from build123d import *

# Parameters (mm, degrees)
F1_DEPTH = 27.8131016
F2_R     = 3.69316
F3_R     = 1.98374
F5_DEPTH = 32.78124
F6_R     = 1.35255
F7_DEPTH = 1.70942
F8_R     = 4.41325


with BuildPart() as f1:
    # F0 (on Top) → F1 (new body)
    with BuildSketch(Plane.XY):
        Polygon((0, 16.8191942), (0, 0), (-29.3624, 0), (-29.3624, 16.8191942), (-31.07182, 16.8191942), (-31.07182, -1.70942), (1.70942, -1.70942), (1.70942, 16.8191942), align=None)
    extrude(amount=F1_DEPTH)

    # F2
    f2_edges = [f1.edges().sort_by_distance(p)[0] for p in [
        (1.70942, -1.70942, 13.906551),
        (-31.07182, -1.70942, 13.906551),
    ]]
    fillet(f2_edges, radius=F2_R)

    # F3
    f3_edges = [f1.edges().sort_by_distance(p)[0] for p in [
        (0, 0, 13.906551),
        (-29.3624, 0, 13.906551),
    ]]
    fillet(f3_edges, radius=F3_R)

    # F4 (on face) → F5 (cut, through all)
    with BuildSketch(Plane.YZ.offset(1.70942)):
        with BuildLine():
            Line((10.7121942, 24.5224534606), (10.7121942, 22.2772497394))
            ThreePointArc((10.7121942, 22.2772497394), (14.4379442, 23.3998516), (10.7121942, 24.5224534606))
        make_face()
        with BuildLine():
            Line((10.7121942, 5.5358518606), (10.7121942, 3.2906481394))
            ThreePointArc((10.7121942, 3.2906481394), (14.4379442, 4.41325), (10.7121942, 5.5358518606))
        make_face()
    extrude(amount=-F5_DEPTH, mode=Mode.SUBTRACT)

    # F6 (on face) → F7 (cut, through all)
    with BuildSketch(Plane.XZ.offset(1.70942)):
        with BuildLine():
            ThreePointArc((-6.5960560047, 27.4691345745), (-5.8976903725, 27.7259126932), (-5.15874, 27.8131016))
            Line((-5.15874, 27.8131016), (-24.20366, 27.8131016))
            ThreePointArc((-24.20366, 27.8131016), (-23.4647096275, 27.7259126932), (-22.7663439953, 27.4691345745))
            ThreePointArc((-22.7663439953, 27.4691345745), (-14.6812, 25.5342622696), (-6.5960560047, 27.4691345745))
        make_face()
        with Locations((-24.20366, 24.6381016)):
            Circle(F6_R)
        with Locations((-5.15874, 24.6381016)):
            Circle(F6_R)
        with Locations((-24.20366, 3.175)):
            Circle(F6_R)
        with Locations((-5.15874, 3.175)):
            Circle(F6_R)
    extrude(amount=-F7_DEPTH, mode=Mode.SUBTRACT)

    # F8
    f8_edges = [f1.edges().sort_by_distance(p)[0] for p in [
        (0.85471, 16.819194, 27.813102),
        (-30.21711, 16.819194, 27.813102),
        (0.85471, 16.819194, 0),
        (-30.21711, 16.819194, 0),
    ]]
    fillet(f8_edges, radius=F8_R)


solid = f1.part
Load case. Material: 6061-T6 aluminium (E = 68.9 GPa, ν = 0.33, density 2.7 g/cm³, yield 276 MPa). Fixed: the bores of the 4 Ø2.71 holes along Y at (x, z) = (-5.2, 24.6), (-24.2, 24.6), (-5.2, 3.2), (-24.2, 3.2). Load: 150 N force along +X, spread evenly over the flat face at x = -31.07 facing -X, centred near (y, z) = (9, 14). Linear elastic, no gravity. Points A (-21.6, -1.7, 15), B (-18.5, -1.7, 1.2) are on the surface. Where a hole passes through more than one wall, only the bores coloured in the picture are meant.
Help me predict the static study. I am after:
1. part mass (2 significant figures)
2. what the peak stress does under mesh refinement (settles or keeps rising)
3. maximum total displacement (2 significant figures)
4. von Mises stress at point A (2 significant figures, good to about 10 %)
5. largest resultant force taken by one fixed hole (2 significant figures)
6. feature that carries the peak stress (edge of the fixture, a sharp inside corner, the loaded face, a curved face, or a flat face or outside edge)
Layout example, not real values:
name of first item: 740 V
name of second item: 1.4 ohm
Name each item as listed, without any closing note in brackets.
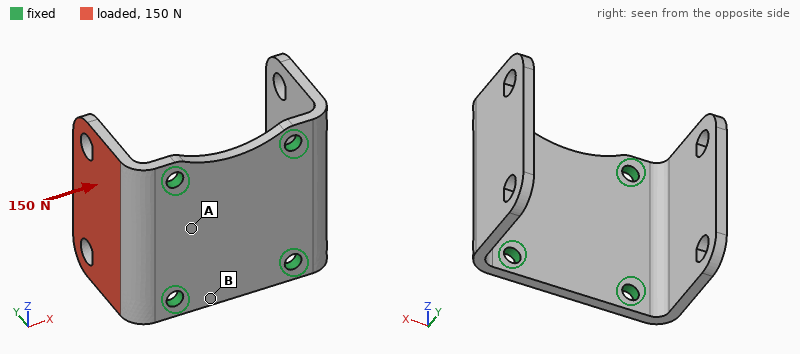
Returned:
part mass: 7.7 g
what the peak stress does under mesh refinement: keeps rising
maximum total displacement: 0.29 mm
von Mises stress at point A: 28 MPa
largest resultant force taken by one fixed hole: 56 N
feature that carries the peak stress: edge of the fixture
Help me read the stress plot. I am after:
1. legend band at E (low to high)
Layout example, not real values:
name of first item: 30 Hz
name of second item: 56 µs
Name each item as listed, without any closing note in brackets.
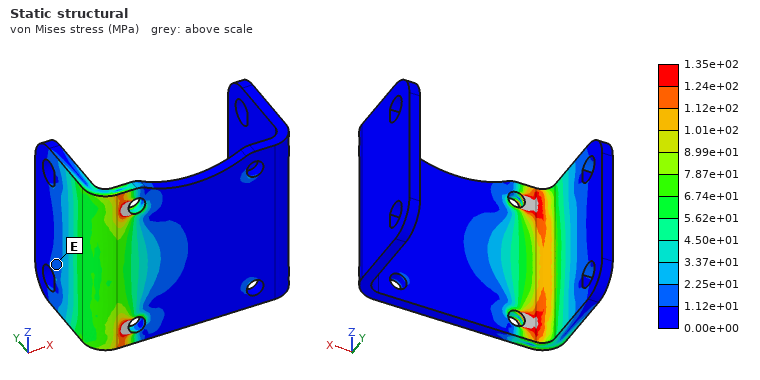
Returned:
legend band at E: 1.12e+01 to 2.25e+01 MPa
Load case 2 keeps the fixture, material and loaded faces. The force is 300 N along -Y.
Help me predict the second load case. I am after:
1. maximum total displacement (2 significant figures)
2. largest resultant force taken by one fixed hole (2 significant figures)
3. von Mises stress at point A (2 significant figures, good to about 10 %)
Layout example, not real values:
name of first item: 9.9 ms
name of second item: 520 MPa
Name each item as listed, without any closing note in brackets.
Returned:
maximum total displacement: 0.18 mm
largest resultant force taken by one fixed hole: 160 N
von Mises stress at point A: 25 MPa
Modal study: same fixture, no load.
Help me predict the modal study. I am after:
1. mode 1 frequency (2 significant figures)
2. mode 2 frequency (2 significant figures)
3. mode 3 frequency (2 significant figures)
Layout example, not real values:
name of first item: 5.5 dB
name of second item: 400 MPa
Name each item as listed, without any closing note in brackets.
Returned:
mode 1 frequency: 3300 Hz
mode 2 frequency: 3400 Hz
mode 3 frequency: 7100 Hz
